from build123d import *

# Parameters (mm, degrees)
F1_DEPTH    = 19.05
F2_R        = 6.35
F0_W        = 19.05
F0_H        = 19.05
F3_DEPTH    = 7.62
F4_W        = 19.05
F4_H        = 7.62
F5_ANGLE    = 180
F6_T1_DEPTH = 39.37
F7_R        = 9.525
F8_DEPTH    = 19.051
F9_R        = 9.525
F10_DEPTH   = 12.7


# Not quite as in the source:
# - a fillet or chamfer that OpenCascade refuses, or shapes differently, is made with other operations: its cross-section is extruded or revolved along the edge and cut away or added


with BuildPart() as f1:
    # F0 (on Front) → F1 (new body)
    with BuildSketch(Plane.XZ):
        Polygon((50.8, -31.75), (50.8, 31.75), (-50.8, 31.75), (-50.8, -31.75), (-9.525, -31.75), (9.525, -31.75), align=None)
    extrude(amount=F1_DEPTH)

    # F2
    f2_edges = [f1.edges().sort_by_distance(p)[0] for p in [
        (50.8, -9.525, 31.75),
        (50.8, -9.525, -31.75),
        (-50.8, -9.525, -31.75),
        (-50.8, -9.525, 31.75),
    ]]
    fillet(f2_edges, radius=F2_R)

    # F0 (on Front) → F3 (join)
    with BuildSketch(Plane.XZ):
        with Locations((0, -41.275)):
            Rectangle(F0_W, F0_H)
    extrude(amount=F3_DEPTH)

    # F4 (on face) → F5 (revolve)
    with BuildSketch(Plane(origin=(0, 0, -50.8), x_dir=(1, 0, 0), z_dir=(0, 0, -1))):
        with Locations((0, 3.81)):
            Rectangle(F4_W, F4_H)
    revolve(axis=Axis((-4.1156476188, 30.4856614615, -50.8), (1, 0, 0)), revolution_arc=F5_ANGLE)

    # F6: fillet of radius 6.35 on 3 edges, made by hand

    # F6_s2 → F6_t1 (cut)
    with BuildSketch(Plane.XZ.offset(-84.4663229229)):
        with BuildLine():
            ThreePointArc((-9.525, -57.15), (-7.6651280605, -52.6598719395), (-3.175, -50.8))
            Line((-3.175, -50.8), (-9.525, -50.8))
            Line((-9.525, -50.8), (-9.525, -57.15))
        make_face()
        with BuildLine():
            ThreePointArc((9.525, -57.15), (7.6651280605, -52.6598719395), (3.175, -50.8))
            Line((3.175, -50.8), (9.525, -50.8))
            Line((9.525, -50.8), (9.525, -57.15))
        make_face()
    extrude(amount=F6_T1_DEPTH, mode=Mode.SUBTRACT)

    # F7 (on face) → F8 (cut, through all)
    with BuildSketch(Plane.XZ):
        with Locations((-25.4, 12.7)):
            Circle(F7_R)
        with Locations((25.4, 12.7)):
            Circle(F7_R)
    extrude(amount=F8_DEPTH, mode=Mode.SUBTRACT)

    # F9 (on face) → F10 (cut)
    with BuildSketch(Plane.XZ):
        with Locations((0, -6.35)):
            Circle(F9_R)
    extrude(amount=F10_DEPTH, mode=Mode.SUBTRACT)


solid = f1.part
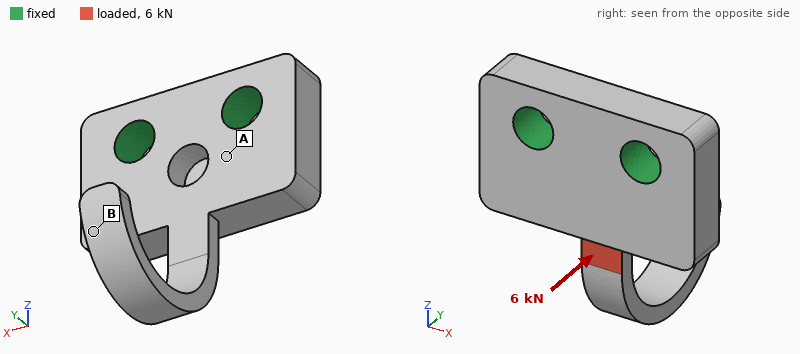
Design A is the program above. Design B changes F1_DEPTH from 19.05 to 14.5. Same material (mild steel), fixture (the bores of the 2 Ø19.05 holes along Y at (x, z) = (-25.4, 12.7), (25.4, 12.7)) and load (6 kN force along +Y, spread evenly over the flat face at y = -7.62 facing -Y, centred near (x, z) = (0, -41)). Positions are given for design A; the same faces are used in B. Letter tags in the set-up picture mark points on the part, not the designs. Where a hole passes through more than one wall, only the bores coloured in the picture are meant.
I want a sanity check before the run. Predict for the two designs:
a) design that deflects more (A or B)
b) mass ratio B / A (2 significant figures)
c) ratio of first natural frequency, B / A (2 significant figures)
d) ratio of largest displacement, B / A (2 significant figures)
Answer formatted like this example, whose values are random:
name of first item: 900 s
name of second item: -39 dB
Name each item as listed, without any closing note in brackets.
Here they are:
design that deflects more: B
mass ratio B / A: 0.79
ratio of first natural frequency, B / A: 0.99
ratio of largest displacement, B / A: 1.3
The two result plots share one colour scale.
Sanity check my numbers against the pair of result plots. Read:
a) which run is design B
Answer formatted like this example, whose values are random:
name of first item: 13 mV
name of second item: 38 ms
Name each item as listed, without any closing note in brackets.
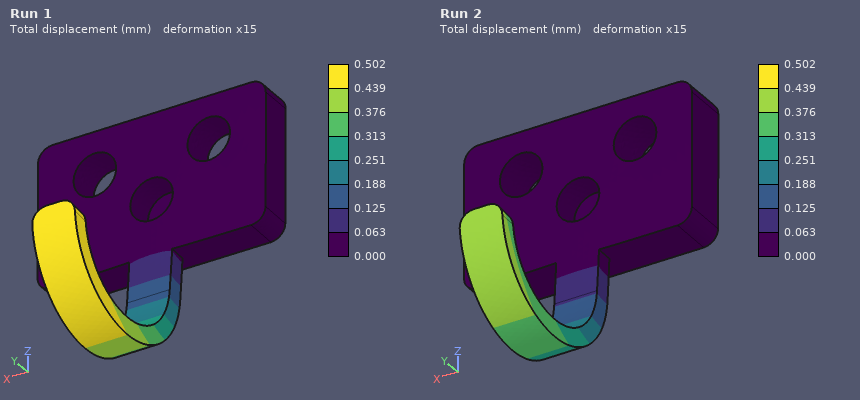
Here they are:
which run is design B: Run 1
